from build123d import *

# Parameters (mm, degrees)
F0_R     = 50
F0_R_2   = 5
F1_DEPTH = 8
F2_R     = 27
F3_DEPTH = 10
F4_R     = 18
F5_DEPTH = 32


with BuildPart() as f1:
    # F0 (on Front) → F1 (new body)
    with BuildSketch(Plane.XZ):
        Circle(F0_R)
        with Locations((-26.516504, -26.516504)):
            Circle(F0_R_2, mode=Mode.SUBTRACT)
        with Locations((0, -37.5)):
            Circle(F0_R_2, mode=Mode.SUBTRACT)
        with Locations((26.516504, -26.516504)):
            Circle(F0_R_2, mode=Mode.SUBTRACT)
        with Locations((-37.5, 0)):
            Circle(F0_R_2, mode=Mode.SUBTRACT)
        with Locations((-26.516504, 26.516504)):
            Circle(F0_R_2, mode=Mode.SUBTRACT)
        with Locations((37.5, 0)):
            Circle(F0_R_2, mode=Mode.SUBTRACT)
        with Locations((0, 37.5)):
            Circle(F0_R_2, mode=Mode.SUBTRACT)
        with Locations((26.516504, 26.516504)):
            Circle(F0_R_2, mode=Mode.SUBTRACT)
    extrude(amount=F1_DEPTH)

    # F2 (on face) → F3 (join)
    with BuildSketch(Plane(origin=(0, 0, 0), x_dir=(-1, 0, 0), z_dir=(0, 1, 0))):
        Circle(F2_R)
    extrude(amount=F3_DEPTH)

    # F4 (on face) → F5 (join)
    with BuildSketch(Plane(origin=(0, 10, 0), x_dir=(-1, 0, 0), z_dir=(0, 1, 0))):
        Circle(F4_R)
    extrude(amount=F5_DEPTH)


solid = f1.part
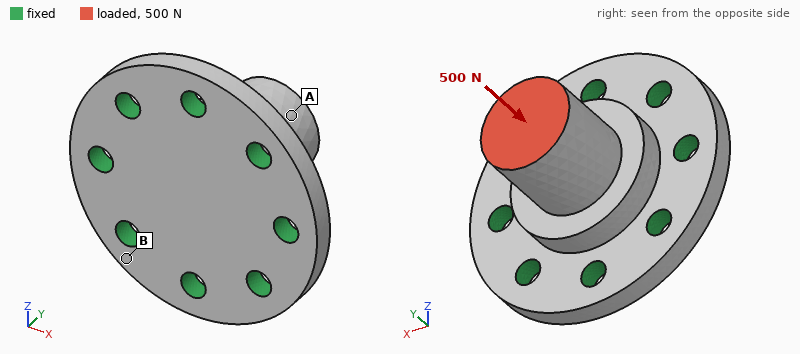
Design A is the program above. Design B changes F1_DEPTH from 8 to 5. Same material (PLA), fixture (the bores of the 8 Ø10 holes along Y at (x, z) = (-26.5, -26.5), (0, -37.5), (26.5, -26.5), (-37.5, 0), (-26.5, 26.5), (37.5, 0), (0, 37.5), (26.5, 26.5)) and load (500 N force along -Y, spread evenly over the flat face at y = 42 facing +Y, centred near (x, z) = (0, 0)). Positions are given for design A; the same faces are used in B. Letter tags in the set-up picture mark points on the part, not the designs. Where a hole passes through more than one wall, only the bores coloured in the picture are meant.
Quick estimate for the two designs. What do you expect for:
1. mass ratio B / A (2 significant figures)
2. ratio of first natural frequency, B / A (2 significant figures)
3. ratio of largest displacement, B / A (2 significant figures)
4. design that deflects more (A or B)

0.81
0.84
1.5
B
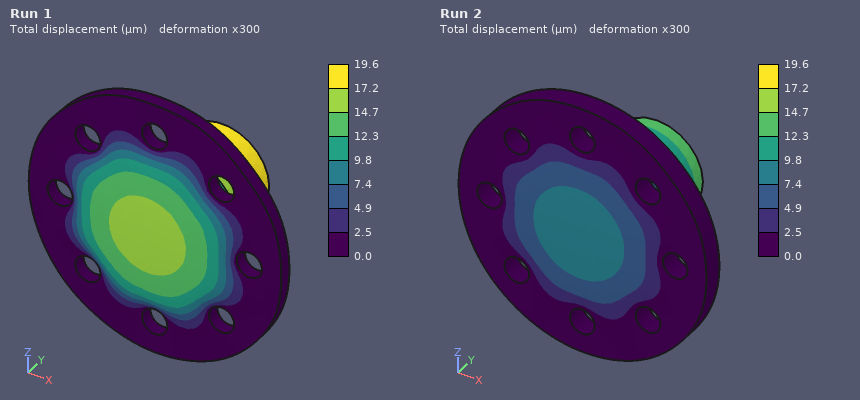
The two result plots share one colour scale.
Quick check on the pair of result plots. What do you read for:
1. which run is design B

Run 1
